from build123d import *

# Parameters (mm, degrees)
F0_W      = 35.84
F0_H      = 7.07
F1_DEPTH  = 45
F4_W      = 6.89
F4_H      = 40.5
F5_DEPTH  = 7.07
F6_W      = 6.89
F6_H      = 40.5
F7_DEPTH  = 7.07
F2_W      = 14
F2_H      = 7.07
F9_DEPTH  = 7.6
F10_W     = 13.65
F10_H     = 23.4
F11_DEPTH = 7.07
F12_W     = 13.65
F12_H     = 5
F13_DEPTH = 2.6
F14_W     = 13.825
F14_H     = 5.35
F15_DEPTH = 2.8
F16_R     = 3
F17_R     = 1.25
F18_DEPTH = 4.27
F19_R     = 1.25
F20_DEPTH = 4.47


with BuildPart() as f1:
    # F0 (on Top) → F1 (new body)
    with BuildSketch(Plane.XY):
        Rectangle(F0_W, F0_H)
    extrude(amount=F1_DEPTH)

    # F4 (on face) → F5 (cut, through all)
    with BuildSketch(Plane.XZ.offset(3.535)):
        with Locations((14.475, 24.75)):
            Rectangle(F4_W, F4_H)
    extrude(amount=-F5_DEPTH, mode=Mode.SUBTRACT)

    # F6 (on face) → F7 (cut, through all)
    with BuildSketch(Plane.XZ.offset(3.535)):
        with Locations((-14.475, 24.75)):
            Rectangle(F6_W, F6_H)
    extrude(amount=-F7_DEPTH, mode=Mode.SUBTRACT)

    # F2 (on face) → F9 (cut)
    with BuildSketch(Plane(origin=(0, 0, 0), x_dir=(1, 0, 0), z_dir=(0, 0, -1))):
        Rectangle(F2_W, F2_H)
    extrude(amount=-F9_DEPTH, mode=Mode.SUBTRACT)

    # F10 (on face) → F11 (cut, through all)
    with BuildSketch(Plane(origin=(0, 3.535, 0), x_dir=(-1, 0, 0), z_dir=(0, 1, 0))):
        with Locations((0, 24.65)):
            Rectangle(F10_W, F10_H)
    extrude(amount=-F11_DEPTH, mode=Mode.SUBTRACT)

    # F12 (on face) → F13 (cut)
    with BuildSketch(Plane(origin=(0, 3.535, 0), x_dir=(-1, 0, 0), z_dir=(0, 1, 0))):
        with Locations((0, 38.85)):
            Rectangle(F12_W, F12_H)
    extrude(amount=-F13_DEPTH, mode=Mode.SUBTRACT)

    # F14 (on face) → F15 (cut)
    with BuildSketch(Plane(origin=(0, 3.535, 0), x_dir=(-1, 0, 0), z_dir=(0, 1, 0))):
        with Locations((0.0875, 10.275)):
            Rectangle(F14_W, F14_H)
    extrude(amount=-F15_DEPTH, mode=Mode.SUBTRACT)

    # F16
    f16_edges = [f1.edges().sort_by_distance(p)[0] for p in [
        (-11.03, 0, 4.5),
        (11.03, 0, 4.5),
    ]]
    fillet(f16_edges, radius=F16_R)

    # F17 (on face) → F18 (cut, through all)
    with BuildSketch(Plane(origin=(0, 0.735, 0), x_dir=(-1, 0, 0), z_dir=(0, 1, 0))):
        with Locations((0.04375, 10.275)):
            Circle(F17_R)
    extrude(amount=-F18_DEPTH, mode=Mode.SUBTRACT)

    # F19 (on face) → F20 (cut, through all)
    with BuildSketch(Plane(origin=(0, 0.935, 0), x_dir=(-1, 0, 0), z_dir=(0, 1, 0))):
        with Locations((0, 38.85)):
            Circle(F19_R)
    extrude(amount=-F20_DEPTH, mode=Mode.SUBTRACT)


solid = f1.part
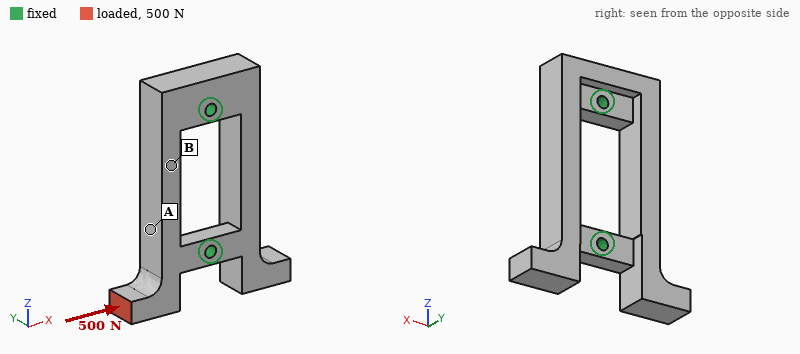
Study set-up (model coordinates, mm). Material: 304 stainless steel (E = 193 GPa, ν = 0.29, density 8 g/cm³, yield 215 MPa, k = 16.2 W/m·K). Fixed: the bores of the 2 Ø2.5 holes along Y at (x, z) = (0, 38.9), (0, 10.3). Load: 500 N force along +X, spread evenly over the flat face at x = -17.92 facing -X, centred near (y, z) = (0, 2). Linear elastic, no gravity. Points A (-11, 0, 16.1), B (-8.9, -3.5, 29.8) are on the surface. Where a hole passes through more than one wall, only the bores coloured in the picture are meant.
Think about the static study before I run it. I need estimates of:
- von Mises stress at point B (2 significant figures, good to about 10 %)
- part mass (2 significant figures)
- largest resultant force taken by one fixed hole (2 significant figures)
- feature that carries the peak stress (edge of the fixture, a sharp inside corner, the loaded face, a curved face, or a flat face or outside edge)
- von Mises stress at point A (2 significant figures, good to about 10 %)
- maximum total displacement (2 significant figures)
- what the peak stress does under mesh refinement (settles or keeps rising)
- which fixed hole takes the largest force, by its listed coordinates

23 MPa
32 g
650 N
a sharp inside corner
53 MPa
41 µm
keeps rising
(0, 10.3)
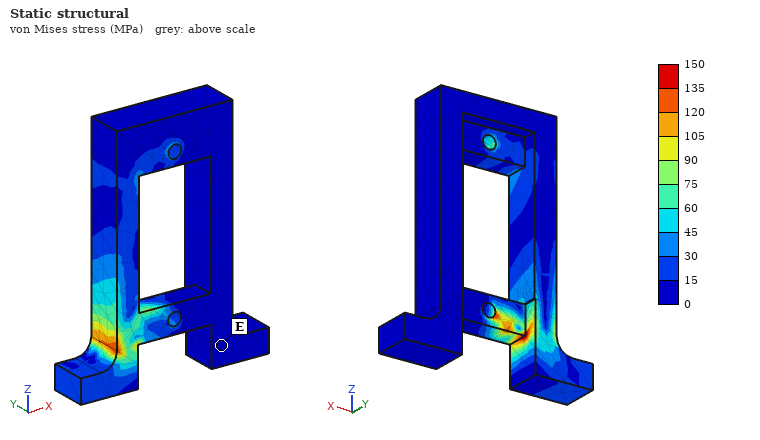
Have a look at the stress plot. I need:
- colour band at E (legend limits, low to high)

0 to 15 MPa
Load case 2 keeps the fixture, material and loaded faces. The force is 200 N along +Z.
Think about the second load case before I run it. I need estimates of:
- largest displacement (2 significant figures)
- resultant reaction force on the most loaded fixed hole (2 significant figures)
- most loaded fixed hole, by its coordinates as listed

28 µm
250 N
(0, 38.9)
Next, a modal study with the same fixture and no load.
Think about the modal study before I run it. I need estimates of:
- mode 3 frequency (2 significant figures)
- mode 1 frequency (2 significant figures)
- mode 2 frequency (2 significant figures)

10 kHz
7300 Hz
7400 Hz
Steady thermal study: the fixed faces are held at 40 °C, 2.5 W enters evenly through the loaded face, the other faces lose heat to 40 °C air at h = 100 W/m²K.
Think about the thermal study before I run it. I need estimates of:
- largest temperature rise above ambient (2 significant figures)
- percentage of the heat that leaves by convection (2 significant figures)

61 K
68 %
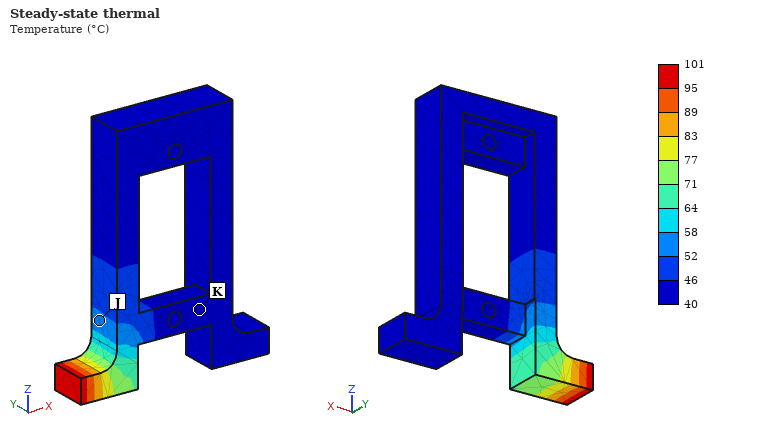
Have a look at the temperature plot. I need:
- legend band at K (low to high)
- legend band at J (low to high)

40 to 46 °C
52 to 58 °C
